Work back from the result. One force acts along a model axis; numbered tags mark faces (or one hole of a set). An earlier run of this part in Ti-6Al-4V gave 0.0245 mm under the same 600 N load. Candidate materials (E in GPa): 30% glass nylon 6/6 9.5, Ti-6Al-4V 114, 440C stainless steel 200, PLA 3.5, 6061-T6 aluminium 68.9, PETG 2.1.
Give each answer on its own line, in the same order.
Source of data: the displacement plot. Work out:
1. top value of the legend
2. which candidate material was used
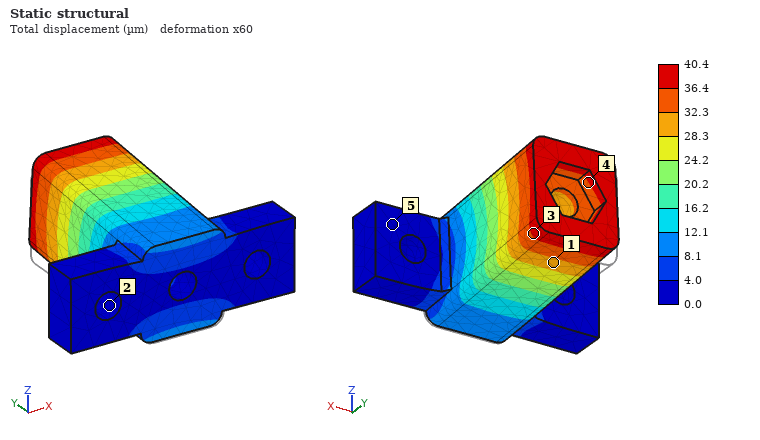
40.4 µm
6061-T6 aluminium
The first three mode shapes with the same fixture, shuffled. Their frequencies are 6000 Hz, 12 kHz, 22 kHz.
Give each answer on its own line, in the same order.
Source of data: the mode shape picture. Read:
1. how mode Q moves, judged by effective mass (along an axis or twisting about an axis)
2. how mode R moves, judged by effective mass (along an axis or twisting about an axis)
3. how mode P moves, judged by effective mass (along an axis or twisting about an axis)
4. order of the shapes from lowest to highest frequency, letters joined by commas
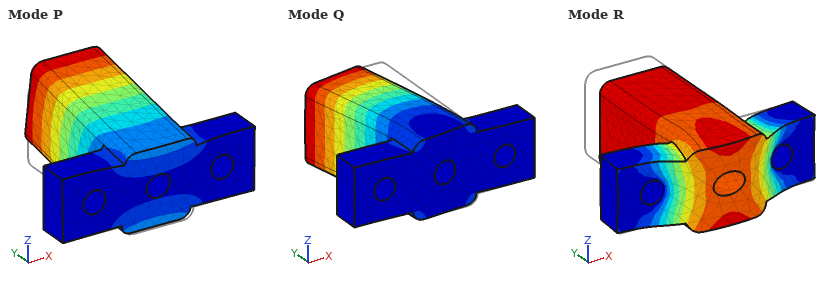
along X
along Y
along Z
P, Q, R
